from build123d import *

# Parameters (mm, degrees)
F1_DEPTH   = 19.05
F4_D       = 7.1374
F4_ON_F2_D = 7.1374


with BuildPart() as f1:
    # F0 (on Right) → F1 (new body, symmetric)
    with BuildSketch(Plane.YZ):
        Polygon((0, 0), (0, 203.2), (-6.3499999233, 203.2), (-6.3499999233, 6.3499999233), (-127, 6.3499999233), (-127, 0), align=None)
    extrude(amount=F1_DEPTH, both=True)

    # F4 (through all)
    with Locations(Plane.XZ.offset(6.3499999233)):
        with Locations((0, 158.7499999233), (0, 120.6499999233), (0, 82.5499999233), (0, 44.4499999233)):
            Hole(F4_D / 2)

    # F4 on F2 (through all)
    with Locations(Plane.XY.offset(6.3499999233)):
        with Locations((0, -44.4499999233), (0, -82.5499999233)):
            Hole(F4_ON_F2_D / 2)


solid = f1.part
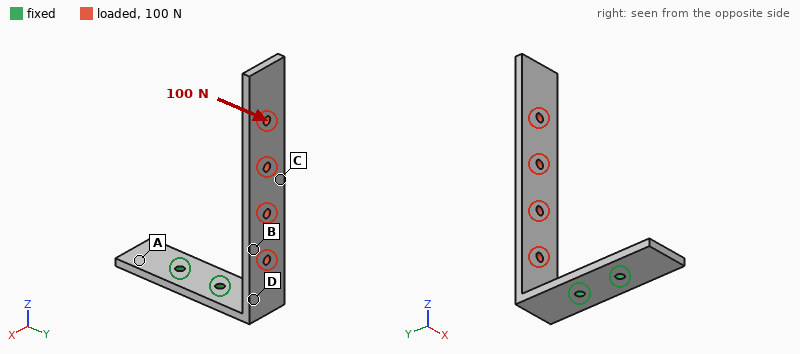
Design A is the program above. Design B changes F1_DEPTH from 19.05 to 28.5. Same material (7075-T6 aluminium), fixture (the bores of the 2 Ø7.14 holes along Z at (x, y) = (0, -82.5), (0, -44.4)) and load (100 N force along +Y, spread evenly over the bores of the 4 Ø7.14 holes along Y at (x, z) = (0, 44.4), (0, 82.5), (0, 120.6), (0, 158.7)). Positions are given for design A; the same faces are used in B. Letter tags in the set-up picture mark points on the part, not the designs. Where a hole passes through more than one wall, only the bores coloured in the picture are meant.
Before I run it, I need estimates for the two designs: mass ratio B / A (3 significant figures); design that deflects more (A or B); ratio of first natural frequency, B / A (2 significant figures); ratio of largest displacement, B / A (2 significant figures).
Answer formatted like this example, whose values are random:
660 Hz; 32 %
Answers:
1.51; A; 1.00; 0.67
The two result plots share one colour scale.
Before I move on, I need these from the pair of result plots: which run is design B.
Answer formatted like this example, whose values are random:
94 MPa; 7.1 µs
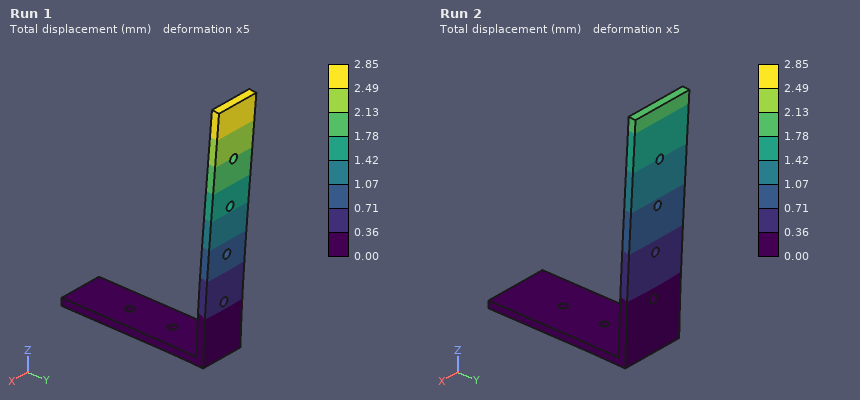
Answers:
Run 2
